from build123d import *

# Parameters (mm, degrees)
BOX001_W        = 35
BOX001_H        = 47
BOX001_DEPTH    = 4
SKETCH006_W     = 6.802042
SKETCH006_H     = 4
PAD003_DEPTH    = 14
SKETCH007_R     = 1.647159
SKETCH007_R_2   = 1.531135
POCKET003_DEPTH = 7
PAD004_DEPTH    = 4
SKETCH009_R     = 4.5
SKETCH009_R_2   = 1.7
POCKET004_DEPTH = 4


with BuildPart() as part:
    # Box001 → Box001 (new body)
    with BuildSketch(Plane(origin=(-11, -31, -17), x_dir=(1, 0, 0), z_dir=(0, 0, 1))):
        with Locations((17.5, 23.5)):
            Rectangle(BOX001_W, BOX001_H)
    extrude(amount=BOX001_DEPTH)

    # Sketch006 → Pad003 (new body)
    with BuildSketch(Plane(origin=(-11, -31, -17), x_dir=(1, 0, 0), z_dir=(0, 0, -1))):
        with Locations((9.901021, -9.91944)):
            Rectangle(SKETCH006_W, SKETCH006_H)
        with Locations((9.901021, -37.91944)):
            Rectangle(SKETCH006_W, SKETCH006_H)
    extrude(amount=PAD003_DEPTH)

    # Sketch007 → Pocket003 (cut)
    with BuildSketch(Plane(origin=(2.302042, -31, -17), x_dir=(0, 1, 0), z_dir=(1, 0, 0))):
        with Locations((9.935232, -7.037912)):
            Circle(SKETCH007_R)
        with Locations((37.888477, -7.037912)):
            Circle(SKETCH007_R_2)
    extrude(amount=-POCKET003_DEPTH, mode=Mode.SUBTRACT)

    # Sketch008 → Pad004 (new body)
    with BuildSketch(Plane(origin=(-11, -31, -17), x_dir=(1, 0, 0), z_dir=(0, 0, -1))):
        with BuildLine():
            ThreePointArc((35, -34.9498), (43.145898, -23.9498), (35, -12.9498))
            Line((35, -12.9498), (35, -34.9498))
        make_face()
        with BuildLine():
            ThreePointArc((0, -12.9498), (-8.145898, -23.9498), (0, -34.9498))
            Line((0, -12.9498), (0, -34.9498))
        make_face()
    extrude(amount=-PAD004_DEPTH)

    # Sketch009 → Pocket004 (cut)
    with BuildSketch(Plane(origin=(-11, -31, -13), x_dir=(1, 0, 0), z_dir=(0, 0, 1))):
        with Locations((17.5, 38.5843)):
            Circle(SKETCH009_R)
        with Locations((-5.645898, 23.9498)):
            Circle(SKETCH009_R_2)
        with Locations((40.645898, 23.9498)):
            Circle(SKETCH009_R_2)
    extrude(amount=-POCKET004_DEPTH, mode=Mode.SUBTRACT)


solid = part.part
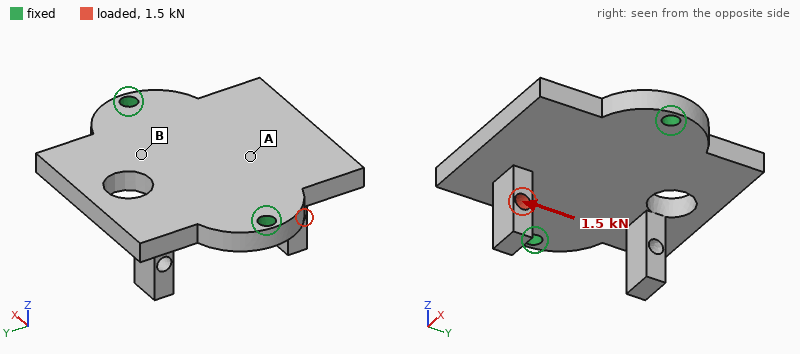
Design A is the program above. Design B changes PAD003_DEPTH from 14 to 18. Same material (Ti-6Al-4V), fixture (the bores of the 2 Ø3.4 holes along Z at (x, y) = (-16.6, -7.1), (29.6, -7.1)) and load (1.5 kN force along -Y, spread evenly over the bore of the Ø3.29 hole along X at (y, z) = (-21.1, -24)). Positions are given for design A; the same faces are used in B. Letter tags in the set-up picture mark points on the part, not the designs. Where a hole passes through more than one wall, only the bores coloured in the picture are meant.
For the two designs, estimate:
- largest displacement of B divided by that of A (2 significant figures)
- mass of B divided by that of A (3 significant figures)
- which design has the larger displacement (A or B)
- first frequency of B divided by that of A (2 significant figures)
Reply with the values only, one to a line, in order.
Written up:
1.2
1.03
B
0.94
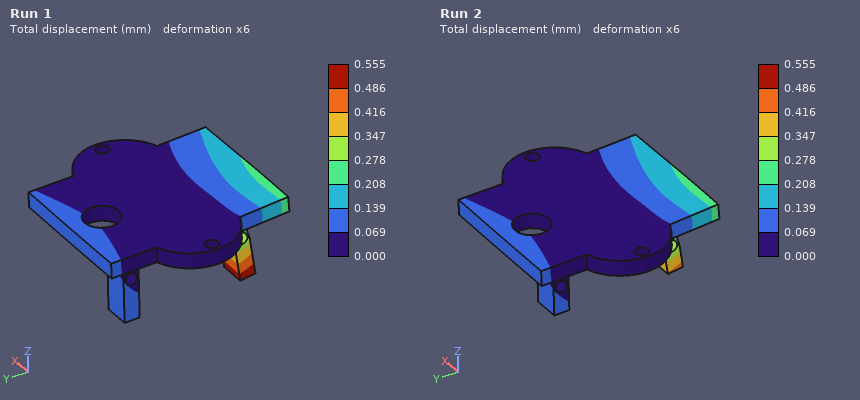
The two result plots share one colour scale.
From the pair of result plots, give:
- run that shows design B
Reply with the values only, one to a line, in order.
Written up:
Run 1
